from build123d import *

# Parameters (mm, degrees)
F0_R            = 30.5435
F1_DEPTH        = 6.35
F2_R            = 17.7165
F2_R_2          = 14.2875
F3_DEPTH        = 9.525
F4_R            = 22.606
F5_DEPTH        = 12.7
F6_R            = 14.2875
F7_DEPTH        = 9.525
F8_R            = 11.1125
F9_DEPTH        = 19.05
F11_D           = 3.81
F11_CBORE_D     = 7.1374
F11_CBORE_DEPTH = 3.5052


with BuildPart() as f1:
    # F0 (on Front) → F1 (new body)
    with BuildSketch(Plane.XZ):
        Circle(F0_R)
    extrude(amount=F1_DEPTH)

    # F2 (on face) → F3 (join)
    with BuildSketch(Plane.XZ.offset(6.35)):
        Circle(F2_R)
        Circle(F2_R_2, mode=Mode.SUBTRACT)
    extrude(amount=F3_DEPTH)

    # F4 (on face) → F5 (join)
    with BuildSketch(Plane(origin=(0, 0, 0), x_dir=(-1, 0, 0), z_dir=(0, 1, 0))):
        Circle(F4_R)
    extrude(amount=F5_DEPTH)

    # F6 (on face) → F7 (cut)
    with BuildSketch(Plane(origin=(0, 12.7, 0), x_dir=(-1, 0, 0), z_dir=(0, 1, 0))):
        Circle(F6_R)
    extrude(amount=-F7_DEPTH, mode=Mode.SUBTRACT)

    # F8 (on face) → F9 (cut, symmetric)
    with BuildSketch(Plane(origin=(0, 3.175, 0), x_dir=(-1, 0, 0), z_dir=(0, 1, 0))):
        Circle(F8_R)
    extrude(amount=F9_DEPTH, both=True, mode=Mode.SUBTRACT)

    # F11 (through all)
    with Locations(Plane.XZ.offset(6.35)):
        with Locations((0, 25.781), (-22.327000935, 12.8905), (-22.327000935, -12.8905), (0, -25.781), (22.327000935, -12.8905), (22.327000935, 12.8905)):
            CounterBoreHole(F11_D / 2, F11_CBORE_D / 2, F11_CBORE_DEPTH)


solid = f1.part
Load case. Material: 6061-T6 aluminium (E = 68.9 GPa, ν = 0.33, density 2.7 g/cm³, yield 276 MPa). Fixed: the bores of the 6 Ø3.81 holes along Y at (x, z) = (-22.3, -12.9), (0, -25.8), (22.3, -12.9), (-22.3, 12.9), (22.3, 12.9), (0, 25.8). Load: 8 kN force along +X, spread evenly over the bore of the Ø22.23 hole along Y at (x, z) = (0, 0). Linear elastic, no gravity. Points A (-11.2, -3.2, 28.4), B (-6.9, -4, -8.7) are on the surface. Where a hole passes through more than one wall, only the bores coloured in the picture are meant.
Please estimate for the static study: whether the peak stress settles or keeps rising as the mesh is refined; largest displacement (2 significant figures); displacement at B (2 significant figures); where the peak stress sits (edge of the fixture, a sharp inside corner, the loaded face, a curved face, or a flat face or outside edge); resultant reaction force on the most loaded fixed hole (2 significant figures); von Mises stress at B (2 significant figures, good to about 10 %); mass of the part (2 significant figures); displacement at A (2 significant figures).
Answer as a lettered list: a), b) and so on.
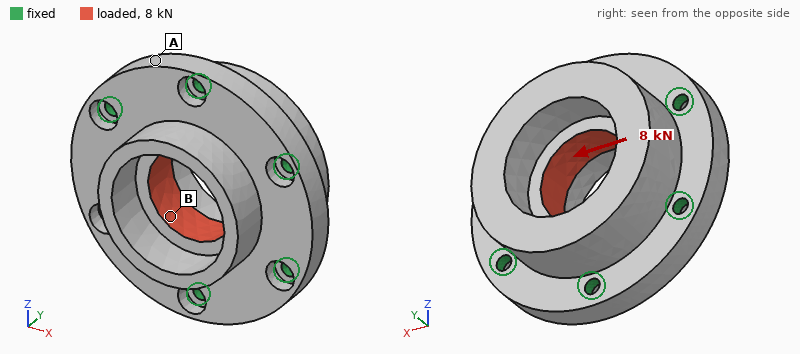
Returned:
a) keeps rising
b) 5.8 µm
c) 5.4 µm
d) edge of the fixture
e) 1.5 kN
f) 18 MPa
g) 85 g
h) 1.8 µm
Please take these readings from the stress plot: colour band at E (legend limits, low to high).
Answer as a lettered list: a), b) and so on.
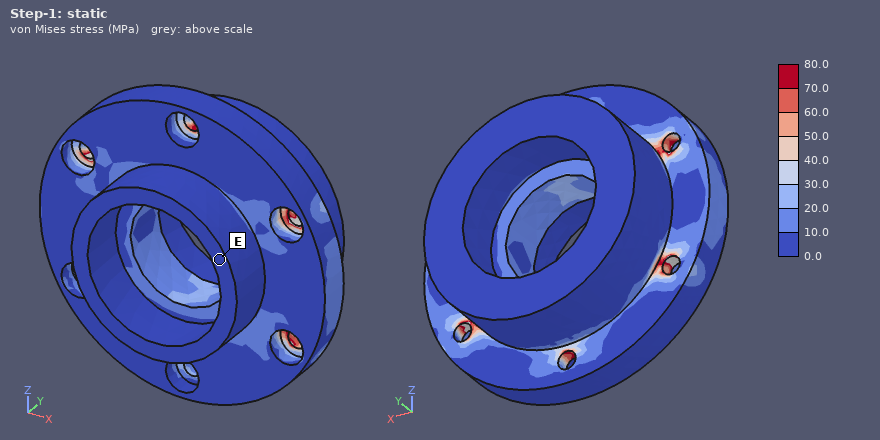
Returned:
a) 0.0 to 10.0 MPa
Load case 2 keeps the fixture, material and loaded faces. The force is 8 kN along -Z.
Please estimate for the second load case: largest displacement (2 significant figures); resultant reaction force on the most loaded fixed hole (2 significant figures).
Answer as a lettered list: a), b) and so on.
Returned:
a) 5.7 µm
b) 1.7 kN
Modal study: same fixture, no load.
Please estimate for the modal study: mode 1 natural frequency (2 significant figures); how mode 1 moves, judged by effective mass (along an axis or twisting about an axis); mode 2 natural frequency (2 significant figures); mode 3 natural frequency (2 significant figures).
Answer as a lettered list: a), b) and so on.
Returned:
a) 18 kHz
b) along Y
c) 21 kHz
d) 21 kHz
